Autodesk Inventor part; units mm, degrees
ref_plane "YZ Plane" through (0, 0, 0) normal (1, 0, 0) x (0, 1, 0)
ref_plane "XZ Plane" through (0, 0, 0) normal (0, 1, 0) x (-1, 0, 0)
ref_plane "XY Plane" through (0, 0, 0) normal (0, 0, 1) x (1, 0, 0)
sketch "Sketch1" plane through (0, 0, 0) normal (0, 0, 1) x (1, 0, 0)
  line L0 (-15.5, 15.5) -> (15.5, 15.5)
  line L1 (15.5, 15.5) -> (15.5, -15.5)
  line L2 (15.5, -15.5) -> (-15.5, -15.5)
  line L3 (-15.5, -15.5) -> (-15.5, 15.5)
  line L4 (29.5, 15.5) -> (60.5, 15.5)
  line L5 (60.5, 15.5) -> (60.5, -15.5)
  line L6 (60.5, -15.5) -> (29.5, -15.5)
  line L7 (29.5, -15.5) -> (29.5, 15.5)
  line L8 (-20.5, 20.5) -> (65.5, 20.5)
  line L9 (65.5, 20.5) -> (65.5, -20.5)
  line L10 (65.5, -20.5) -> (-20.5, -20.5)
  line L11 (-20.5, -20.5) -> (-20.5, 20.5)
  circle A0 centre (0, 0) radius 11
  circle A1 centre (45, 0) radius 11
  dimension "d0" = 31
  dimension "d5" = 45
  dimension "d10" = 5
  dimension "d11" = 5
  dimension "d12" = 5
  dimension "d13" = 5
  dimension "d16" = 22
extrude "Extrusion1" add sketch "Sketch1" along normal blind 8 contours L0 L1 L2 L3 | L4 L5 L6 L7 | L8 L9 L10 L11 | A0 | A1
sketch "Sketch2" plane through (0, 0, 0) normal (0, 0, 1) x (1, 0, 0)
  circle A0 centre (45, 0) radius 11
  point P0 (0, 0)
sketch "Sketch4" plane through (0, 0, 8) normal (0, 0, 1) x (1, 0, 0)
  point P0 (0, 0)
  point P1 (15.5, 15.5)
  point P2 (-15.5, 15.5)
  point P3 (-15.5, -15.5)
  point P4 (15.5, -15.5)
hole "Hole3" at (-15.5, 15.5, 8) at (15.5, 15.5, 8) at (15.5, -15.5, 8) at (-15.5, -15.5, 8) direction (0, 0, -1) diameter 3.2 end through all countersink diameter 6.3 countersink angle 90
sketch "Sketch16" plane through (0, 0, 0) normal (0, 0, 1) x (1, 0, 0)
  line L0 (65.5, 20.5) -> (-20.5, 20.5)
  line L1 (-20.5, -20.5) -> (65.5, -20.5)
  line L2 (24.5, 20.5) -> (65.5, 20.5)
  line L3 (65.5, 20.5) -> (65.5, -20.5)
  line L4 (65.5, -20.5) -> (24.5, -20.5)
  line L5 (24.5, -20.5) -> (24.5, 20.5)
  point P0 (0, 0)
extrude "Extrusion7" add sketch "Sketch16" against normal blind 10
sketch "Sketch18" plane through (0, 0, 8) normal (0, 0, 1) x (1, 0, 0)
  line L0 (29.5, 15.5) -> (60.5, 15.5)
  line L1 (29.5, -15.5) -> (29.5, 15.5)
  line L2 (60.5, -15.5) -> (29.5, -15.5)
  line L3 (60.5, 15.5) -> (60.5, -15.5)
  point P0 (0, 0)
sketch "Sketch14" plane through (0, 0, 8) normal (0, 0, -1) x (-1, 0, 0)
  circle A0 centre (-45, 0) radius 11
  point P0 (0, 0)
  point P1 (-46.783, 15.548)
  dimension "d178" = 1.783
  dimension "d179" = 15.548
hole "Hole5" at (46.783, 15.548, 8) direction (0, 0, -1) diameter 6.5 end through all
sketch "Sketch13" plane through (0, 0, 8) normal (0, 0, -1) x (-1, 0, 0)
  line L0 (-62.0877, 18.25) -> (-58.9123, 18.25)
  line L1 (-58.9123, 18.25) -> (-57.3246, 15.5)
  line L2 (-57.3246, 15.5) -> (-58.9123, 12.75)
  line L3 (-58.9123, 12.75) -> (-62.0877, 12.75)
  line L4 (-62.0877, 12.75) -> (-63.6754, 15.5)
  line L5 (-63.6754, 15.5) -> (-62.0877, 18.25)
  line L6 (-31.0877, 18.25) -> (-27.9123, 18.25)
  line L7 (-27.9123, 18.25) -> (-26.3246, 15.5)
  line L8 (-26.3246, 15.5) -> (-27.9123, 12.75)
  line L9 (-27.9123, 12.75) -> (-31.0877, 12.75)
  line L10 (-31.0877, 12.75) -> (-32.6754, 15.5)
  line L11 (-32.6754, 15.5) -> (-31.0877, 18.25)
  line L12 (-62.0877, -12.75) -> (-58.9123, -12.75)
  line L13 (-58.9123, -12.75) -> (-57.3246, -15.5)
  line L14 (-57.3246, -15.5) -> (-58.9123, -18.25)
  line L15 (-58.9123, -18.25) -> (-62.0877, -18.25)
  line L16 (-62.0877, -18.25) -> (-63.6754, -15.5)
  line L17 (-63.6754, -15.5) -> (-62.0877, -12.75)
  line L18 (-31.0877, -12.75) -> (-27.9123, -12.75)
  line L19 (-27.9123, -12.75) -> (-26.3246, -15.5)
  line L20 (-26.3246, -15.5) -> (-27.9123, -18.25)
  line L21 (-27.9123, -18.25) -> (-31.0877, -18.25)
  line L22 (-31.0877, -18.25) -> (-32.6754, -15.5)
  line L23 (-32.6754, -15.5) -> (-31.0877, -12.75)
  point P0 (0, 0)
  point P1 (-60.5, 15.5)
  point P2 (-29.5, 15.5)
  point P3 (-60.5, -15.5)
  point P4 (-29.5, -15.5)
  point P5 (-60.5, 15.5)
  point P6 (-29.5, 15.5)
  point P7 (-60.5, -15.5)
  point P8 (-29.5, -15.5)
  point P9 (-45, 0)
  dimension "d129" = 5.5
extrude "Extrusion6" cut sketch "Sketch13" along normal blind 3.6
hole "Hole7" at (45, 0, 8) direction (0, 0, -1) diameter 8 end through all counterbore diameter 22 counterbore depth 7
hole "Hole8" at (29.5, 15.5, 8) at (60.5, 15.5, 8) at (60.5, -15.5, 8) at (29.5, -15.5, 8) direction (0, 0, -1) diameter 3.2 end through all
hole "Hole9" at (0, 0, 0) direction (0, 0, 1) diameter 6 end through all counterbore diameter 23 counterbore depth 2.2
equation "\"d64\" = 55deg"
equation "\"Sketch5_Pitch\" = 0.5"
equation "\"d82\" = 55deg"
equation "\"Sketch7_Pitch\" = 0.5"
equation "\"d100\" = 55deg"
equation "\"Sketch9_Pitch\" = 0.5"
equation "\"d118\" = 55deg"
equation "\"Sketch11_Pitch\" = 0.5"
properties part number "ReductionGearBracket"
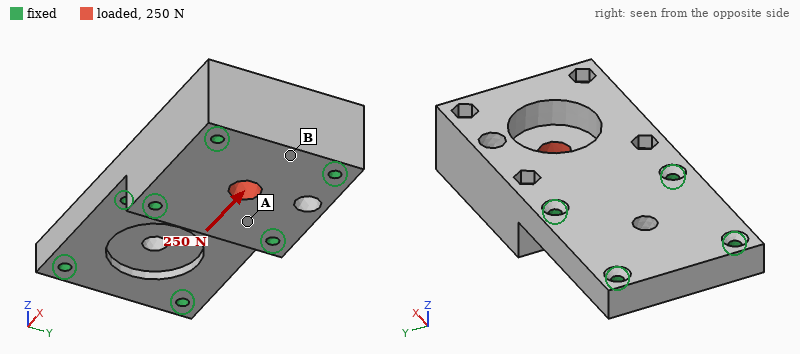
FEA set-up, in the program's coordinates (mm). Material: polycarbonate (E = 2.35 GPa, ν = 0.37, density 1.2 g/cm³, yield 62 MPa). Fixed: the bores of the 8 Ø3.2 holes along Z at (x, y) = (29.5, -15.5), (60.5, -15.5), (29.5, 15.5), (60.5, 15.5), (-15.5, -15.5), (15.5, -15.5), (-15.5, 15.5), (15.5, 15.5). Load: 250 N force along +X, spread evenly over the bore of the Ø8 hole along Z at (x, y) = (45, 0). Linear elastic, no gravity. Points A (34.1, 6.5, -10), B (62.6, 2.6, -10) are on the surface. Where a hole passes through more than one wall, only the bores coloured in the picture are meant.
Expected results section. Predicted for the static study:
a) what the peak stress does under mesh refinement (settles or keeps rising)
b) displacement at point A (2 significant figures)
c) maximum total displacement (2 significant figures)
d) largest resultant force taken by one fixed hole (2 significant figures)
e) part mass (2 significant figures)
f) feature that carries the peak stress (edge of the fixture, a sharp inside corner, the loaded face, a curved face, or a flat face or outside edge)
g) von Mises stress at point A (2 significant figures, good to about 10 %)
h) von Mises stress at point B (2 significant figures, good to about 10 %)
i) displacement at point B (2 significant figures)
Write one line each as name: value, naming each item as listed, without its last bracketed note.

what the peak stress does under mesh refinement: keeps rising
displacement at point A: 3.2 µm
maximum total displacement: 6.3 µm
largest resultant force taken by one fixed hole: 66 N
part mass: 47 g
feature that carries the peak stress: edge of the fixture
von Mises stress at point A: 0.51 MPa
von Mises stress at point B: 0.17 MPa
displacement at point B: 4.1 µm
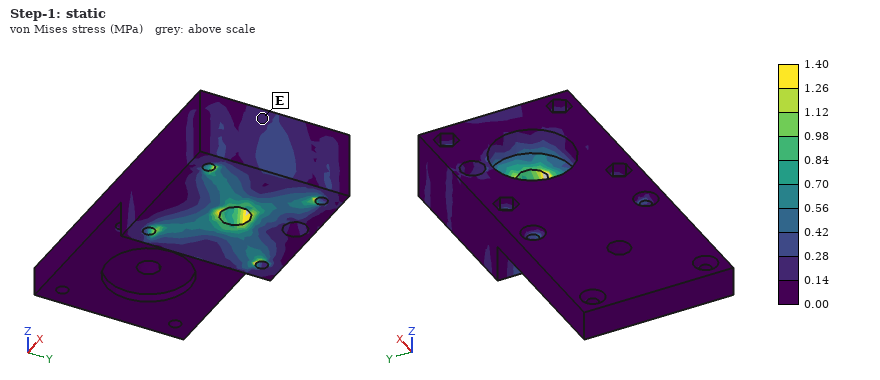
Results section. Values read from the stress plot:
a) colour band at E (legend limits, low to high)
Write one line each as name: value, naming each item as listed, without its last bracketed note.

colour band at E: 0.14 to 0.28 MPa
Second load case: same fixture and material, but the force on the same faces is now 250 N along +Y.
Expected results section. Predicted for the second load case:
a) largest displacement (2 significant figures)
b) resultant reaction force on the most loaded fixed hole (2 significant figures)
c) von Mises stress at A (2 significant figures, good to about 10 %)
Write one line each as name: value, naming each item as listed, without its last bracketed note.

largest displacement: 6.7 µm
resultant reaction force on the most loaded fixed hole: 70 N
von Mises stress at A: 0.46 MPa
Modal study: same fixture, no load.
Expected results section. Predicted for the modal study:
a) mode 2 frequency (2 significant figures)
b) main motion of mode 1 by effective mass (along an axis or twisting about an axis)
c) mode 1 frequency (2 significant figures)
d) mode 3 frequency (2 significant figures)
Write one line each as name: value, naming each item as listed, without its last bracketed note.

mode 2 frequency: 8400 Hz
main motion of mode 1 by effective mass: along Z
mode 1 frequency: 6200 Hz
mode 3 frequency: 8600 Hz
